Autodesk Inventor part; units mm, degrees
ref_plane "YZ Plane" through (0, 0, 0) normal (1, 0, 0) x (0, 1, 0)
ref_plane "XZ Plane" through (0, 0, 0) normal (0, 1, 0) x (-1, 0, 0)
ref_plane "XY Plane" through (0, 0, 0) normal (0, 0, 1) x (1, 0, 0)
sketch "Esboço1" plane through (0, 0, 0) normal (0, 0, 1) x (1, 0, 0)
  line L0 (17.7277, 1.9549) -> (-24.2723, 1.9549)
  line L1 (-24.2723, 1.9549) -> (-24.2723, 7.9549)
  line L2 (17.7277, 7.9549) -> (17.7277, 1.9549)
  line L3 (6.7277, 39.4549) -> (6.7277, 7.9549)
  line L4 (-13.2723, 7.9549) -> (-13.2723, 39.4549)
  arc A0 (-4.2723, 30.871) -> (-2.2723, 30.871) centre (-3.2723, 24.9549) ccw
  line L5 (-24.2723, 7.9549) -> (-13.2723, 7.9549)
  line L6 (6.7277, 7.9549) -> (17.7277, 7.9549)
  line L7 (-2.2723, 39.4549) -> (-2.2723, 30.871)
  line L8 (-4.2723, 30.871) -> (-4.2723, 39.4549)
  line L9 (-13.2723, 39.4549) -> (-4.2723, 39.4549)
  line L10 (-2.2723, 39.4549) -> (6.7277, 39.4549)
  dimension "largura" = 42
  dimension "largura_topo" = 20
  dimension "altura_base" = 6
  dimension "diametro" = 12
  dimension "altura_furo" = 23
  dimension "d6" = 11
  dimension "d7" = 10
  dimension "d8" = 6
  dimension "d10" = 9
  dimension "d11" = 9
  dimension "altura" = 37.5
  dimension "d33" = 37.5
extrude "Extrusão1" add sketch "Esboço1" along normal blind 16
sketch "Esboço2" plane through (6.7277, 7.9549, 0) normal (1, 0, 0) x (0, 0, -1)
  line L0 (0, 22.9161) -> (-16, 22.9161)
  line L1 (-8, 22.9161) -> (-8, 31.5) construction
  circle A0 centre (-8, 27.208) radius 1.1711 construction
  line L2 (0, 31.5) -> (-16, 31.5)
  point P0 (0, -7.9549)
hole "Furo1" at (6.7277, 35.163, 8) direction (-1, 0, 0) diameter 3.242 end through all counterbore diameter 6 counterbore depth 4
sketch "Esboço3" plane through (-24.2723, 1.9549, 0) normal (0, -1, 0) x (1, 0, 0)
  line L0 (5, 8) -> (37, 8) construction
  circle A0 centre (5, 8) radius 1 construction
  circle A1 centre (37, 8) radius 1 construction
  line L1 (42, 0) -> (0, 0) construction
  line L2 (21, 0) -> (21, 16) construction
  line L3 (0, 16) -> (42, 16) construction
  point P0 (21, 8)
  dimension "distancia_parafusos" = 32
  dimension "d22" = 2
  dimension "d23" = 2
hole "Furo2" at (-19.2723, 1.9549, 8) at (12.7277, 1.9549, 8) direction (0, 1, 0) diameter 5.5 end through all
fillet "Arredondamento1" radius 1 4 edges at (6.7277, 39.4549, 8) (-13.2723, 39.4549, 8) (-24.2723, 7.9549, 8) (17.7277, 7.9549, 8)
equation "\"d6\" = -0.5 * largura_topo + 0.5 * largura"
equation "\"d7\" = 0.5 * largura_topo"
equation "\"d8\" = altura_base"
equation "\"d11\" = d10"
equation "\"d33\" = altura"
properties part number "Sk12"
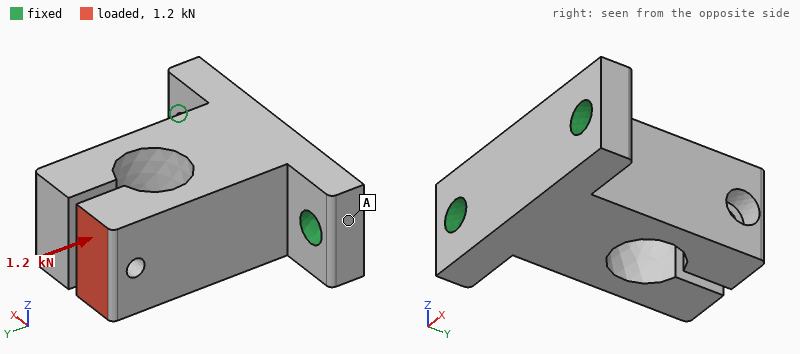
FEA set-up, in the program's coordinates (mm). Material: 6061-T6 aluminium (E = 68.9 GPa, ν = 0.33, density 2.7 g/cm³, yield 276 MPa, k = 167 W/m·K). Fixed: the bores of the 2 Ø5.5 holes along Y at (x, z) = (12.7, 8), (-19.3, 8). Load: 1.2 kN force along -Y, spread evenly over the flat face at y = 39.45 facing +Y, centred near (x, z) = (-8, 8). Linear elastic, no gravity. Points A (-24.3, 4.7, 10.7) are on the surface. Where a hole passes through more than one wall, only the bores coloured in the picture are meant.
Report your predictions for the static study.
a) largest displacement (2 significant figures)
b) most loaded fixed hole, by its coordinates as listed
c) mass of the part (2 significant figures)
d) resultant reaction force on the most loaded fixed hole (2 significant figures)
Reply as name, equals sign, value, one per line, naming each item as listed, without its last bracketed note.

largest displacement = 73 µm
most loaded fixed hole, by its coordinates as listed = (-19.3, 8)
mass of the part = 31 g
resultant reaction force on the most loaded fixed hole = 870 N
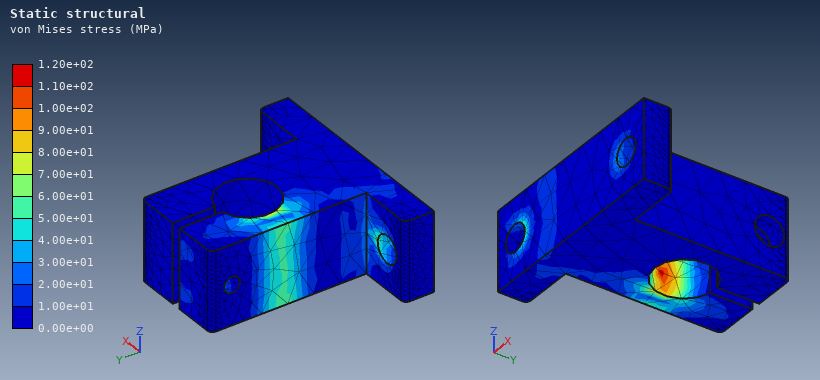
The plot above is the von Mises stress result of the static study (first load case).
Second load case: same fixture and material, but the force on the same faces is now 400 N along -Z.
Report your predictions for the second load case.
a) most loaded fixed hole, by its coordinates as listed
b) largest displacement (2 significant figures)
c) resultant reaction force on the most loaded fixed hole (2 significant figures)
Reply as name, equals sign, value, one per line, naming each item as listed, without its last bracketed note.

most loaded fixed hole, by its coordinates as listed = (-19.3, 8)
largest displacement = 96 µm
resultant reaction force on the most loaded fixed hole = 250 N
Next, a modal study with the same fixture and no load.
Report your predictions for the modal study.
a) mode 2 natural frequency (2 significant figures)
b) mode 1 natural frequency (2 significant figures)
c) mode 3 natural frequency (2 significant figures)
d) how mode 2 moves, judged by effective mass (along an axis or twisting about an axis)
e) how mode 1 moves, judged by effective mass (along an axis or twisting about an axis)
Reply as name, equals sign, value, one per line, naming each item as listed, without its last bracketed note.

mode 2 natural frequency = 5500 Hz
mode 1 natural frequency = 4400 Hz
mode 3 natural frequency = 6000 Hz
how mode 2 moves, judged by effective mass = along X
how mode 1 moves, judged by effective mass = along Z
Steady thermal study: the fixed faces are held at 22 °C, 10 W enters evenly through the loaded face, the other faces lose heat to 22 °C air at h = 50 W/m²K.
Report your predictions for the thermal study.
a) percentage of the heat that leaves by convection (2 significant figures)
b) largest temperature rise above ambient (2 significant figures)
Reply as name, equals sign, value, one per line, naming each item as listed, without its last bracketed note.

percentage of the heat that leaves by convection = 11 %
largest temperature rise above ambient = 20 K
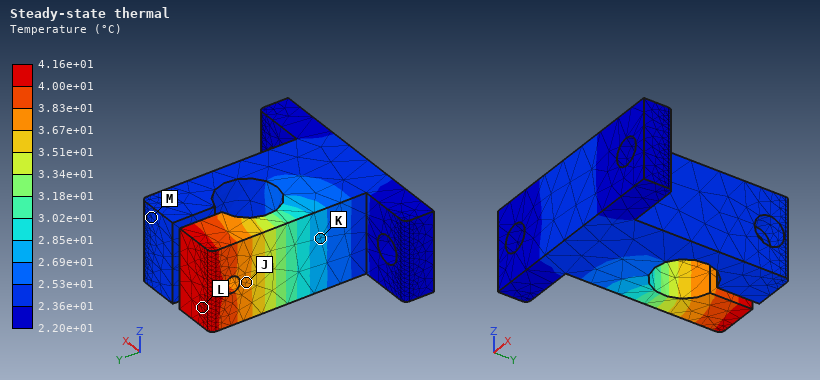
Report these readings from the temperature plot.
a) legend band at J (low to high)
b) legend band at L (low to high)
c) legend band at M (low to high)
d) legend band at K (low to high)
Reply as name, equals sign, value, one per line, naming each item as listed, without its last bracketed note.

legend band at J = 3.67e+01 to 3.83e+01 °C
legend band at L = 4.00e+01 to 4.16e+01 °C
legend band at M = 2.36e+01 to 2.53e+01 °C
legend band at K = 2.69e+01 to 2.85e+01 °C
